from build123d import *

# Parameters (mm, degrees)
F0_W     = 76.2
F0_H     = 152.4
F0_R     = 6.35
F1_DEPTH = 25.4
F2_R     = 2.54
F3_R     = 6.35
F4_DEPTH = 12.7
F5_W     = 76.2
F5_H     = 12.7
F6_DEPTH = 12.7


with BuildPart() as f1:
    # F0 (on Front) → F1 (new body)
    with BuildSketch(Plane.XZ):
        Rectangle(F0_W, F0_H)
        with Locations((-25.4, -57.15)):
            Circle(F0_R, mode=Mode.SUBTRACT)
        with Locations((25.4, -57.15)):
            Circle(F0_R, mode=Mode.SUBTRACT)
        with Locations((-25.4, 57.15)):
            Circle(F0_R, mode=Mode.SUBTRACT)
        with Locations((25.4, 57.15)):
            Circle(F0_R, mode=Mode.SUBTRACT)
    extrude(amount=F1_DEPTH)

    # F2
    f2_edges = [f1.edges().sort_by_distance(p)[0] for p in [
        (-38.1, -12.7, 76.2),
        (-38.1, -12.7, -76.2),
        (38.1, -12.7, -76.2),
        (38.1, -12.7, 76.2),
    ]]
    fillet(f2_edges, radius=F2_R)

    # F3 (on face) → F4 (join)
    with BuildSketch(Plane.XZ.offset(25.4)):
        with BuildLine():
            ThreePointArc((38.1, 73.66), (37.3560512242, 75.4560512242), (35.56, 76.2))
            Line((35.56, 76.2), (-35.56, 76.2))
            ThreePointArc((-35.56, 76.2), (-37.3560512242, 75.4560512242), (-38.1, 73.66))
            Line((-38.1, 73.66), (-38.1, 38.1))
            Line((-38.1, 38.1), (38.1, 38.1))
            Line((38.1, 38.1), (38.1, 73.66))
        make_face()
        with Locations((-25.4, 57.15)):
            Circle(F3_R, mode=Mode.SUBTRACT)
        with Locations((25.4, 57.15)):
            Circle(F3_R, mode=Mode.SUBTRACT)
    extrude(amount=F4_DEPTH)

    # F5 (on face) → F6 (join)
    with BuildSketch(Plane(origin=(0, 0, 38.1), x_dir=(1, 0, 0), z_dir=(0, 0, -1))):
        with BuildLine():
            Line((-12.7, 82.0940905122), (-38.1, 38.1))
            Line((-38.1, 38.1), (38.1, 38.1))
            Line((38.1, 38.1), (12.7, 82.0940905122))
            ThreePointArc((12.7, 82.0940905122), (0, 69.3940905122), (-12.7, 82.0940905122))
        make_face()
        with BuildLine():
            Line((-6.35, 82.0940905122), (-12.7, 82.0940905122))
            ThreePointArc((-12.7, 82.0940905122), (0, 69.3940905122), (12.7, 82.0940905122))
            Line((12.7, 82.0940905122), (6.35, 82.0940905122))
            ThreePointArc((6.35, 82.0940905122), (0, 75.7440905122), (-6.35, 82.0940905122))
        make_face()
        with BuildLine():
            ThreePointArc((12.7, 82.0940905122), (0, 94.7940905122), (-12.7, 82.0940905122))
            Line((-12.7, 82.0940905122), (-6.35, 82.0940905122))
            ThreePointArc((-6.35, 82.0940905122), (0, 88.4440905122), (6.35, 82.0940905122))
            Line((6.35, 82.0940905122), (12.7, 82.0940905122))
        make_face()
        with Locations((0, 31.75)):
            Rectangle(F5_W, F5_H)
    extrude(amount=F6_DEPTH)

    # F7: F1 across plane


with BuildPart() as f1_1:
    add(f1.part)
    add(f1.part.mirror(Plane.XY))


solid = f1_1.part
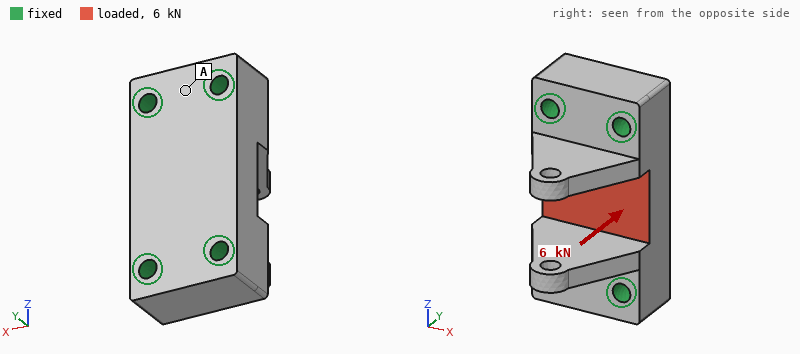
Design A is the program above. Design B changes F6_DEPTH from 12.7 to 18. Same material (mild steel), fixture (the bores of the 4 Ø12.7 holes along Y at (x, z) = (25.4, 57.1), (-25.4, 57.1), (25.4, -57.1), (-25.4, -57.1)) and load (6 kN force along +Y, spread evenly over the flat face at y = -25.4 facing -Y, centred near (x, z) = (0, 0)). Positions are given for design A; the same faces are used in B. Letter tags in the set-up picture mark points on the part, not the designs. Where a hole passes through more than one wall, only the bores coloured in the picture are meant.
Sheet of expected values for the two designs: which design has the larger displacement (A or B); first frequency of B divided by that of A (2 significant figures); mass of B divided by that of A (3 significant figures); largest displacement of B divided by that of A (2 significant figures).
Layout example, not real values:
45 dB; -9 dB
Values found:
B; 1.2; 1.08; 1.2
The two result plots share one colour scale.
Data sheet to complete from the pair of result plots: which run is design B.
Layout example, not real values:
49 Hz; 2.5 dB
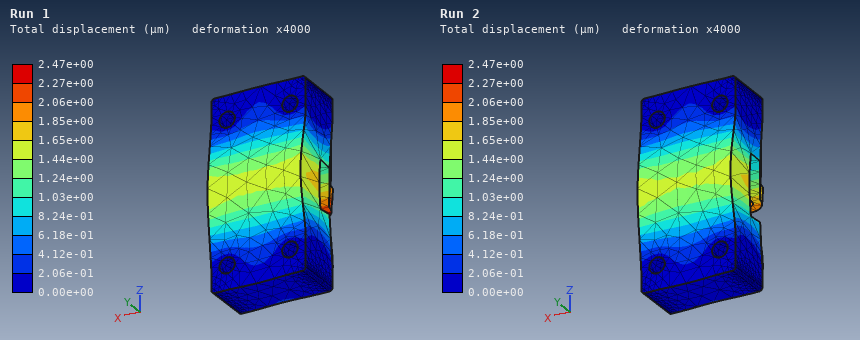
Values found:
Run 1
